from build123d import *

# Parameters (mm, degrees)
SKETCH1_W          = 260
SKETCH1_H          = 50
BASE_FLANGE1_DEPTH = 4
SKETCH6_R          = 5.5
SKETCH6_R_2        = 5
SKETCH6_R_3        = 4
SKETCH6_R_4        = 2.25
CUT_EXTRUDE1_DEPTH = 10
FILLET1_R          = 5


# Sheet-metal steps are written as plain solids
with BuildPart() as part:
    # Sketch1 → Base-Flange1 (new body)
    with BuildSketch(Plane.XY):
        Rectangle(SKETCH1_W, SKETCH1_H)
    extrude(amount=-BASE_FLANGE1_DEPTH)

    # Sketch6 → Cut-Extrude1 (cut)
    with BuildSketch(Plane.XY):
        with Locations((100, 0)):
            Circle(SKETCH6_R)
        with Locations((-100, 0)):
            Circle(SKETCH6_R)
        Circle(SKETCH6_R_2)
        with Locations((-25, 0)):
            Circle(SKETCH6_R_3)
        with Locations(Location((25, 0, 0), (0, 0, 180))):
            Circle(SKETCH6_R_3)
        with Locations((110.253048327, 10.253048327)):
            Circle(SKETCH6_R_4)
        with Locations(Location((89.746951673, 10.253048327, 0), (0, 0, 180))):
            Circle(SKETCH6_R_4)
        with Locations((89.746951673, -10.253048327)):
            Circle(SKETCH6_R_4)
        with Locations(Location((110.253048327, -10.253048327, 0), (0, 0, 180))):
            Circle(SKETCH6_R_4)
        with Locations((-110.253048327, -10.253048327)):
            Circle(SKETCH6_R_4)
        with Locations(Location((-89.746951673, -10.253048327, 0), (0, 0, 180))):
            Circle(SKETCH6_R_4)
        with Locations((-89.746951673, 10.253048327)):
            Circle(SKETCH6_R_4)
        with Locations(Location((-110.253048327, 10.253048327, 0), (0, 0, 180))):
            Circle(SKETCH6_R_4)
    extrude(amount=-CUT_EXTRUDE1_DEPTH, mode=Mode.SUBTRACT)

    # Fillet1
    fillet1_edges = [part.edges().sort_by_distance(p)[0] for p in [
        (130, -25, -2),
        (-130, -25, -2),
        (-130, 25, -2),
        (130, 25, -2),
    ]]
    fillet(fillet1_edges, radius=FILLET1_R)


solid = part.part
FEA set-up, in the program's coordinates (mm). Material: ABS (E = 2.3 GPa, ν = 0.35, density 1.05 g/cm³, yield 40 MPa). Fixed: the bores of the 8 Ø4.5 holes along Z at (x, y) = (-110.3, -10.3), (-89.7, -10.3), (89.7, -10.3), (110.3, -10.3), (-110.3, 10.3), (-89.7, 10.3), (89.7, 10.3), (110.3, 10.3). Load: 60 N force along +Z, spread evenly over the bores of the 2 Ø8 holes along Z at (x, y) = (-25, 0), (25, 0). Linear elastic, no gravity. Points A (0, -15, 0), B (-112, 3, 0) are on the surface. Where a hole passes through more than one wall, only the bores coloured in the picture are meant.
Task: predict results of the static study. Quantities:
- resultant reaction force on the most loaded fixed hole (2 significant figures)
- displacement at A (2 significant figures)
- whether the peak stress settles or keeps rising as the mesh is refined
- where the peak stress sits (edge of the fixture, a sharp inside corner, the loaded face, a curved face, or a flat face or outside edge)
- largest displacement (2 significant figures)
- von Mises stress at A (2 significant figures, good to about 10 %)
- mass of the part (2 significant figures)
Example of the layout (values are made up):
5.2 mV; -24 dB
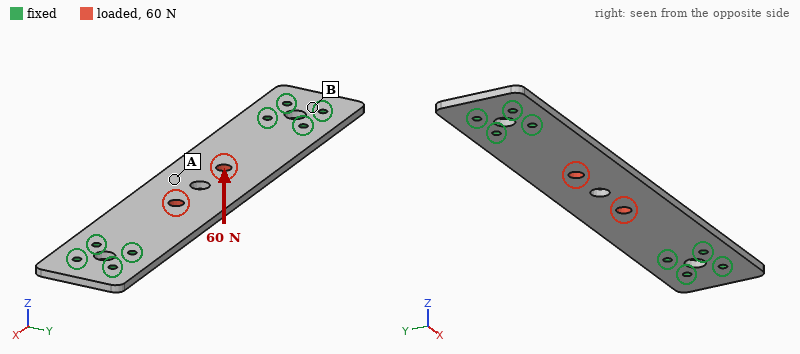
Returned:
23 N; 2.4 mm; keeps rising; edge of the fixture; 2.4 mm; 5.7 MPa; 52 g
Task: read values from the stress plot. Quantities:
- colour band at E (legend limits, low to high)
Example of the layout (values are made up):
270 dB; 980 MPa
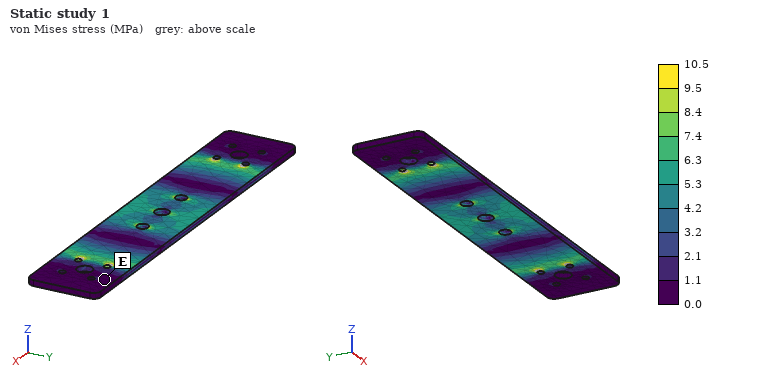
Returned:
0.0 to 1.1 MPa
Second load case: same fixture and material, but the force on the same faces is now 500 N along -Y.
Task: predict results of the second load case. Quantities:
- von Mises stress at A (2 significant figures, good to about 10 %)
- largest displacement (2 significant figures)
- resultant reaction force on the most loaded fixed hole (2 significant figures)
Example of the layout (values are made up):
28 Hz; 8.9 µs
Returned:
2.3 MPa; 0.29 mm; 280 N
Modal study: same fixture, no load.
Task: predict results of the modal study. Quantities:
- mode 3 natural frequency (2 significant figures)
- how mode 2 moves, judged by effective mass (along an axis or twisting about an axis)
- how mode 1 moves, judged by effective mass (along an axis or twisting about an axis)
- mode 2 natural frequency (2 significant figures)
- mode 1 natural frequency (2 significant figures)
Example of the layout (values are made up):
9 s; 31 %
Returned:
520 Hz; twisting about X; along Z; 450 Hz; 190 Hz
